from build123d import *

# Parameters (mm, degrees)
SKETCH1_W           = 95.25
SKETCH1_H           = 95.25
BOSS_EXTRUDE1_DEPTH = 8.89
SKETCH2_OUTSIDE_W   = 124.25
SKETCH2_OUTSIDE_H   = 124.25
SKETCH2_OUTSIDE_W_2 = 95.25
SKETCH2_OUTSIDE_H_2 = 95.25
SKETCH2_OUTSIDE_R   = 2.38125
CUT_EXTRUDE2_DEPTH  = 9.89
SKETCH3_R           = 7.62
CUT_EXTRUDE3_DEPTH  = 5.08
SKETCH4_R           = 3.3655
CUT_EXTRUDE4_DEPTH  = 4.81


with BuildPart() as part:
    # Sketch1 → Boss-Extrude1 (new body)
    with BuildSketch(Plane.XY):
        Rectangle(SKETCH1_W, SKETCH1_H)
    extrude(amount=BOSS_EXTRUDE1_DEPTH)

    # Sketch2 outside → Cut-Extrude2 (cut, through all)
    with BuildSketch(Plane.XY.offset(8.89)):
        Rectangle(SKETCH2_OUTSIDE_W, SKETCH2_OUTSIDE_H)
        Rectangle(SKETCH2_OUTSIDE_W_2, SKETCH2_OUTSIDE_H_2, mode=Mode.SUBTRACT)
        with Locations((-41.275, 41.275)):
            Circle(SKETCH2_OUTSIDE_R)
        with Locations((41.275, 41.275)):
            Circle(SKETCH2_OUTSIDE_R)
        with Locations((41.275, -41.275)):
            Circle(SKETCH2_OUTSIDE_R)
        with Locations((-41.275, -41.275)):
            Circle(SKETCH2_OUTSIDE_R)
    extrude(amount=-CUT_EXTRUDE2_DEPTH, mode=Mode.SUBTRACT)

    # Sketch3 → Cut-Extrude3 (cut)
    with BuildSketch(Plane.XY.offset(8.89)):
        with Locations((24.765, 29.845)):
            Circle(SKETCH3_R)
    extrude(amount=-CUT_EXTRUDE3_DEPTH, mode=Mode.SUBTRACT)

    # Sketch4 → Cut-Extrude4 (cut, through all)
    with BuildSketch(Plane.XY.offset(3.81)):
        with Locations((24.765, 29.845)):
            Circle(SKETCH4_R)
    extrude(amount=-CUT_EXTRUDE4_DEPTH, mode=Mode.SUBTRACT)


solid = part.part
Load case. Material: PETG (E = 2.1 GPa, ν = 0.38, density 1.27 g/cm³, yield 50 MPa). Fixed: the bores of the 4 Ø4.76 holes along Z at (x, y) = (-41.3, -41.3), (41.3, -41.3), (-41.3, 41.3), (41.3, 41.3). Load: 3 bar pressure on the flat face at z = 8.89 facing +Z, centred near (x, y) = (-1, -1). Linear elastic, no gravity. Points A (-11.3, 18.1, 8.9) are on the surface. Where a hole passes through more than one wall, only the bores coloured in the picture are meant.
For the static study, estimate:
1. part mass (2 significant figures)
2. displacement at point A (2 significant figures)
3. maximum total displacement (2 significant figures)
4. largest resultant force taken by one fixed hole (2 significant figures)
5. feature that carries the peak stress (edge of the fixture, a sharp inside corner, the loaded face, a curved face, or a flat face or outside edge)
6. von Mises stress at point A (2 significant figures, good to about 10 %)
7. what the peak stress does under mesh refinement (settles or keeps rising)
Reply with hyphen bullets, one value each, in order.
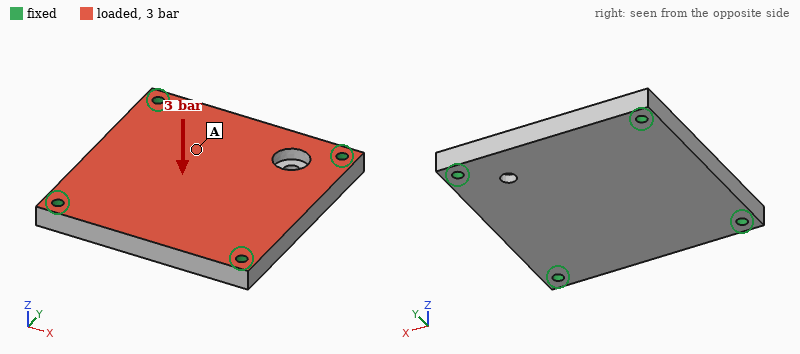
- 100 g
- 0.77 mm
- 0.92 mm
- 670 N
- edge of the fixture
- 7.7 MPa
- keeps rising
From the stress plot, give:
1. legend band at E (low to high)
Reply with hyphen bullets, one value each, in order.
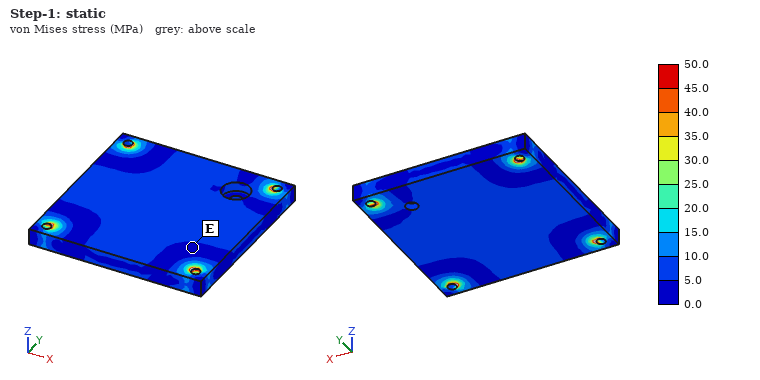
- 0.0 to 5.0 MPa
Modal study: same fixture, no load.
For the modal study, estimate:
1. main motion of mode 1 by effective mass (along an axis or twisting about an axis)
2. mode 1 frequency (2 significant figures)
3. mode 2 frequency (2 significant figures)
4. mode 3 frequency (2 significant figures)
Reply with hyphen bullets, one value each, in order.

- along Z
- 1000 Hz
- 1700 Hz
- 1700 Hz
